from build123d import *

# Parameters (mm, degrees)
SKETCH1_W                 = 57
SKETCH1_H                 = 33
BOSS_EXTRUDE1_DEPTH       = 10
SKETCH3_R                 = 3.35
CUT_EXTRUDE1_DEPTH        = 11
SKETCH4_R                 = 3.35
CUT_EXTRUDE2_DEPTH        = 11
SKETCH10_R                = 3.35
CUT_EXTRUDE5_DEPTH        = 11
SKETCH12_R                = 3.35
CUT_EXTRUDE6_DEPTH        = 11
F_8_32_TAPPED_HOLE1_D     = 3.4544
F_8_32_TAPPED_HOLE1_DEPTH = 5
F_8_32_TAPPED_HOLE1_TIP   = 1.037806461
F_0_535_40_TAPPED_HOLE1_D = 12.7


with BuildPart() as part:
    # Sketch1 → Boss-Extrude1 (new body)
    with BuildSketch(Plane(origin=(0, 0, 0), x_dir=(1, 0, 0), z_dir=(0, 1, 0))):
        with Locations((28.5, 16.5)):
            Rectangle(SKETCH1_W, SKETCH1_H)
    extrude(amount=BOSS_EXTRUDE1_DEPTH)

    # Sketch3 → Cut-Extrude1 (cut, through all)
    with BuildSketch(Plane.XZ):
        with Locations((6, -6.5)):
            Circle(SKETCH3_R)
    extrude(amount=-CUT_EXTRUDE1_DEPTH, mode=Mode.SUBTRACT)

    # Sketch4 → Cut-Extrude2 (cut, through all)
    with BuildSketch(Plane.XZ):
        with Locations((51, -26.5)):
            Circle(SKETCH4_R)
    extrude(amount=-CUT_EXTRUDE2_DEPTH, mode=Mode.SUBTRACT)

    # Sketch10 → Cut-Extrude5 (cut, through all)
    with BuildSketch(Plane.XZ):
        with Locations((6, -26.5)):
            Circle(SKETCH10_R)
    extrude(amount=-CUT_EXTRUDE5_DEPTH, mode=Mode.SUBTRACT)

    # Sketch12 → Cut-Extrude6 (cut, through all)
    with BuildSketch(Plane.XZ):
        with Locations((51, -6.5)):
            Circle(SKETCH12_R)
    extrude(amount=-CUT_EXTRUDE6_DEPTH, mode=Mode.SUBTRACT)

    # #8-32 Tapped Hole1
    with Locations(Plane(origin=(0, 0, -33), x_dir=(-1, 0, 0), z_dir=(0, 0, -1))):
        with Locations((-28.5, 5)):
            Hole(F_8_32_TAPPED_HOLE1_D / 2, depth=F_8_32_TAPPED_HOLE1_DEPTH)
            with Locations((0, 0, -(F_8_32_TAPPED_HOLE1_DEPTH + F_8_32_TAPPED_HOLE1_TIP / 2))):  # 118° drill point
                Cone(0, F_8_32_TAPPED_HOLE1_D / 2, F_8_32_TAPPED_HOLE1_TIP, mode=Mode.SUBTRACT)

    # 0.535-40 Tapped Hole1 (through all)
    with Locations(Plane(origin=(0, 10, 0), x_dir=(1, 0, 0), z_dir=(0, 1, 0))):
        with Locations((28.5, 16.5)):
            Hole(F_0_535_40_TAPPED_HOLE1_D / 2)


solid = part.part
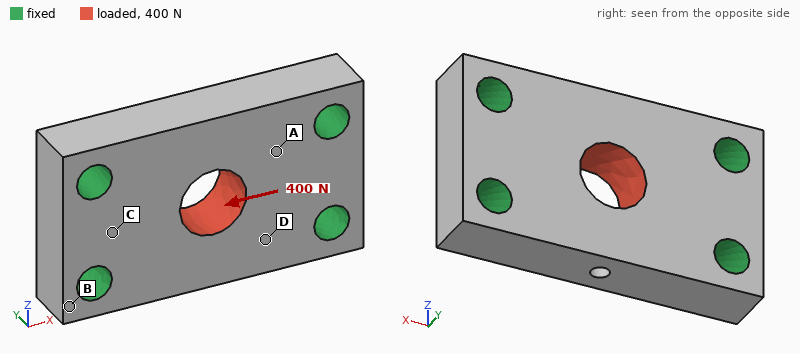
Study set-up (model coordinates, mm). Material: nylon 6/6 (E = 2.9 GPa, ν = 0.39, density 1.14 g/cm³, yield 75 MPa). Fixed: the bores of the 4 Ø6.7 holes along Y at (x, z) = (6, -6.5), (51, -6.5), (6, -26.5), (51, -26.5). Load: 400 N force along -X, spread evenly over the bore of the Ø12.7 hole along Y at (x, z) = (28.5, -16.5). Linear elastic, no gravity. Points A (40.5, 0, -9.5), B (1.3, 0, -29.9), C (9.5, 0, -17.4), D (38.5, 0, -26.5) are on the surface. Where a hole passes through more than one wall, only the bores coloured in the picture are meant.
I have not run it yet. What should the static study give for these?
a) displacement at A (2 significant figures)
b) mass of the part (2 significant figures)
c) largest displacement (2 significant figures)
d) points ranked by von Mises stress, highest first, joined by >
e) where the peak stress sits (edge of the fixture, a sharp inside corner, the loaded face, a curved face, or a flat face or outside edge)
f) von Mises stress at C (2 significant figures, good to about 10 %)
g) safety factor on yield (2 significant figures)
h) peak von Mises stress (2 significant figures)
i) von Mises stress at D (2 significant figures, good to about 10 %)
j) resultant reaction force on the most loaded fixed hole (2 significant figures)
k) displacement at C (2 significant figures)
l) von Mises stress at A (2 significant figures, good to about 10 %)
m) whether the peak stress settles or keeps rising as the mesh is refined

2.4 µm
18 g
5.6 µm
A > D > C > B
the loaded face
0.32 MPa
44
1.7 MPa
0.64 MPa
100 N
1.8 µm
0.88 MPa
settles
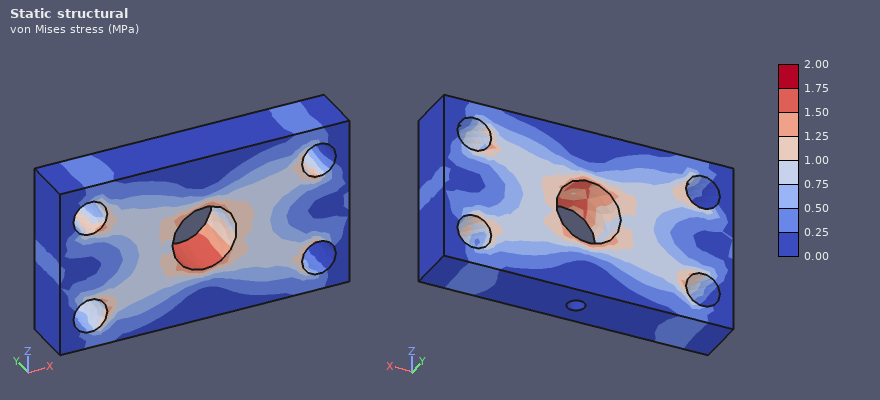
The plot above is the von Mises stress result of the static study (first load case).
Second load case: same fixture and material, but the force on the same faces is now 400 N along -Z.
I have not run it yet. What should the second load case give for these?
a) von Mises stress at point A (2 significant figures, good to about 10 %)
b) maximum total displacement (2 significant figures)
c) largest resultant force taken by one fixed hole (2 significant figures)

1.3 MPa
15 µm
130 N
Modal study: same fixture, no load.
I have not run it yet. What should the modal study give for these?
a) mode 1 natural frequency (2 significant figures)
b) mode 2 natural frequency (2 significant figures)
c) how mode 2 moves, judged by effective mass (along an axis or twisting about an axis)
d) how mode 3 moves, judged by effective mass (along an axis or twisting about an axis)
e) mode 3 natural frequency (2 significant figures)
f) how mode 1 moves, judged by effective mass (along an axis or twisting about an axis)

7400 Hz
8600 Hz
twisting about X
along Z
11 kHz
along Y
